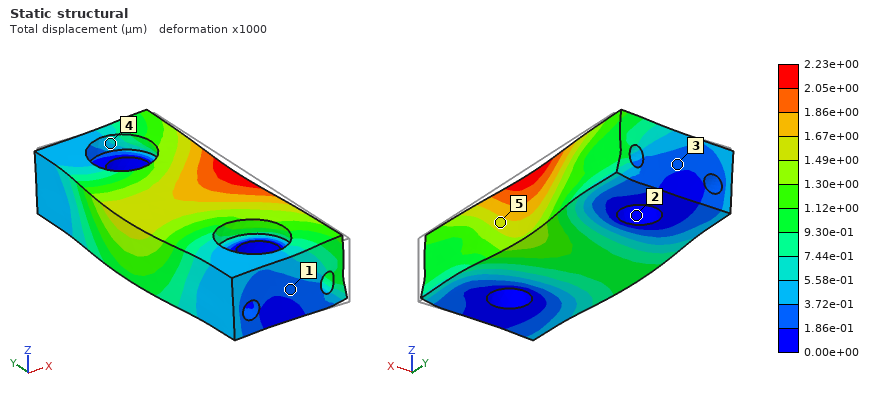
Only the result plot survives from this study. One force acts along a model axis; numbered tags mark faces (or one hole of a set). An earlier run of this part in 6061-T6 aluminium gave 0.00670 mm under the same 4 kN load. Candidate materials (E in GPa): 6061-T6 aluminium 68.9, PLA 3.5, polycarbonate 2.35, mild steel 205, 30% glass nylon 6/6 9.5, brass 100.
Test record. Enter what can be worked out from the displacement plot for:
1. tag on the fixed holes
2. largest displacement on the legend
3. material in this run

2
2.23e+00 µm
mild steel
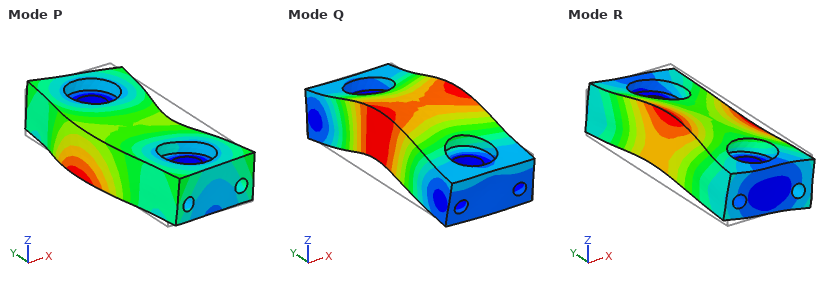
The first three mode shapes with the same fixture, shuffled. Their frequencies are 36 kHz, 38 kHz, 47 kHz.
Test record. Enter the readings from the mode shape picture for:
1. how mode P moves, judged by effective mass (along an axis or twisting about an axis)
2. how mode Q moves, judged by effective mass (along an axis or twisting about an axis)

along X
along Z
